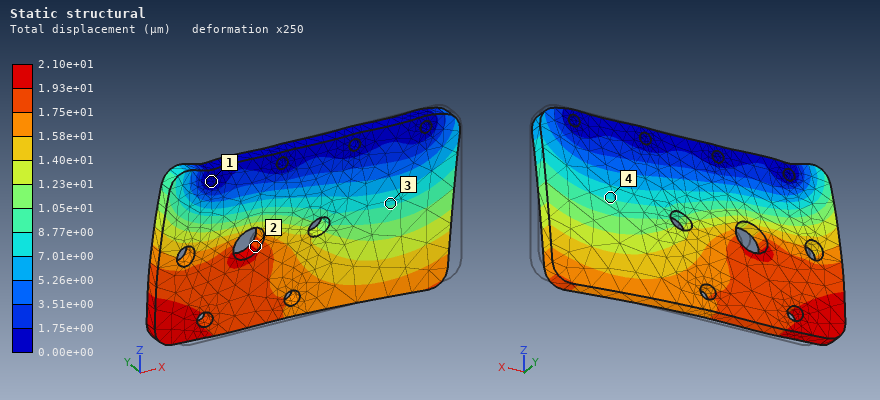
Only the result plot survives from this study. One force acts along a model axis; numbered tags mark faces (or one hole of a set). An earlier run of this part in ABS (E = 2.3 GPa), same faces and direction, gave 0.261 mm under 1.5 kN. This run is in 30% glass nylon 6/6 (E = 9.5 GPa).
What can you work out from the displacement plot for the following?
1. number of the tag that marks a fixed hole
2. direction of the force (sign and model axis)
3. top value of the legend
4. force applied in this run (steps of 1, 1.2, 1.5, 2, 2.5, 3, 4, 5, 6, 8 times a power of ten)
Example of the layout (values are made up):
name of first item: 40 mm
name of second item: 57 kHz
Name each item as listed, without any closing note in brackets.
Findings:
number of the tag that marks a fixed hole: 1
direction of the force: -X
top value of the legend: 2.10e+01 µm
force applied in this run: 500 N
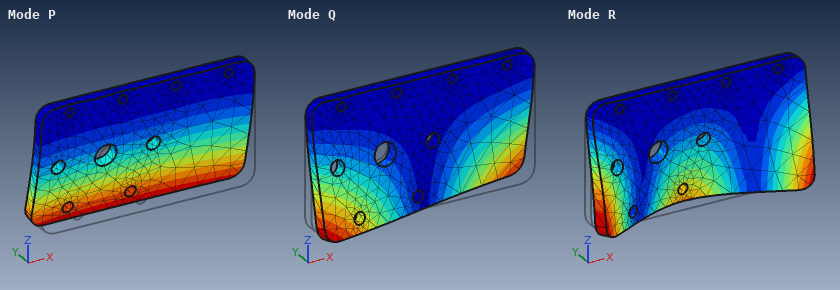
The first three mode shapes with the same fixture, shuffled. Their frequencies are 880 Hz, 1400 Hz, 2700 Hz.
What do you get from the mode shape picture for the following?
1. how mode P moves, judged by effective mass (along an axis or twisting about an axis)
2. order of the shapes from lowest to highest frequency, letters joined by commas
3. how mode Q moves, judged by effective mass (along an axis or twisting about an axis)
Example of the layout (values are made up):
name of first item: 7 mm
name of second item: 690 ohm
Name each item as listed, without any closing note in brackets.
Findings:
how mode P moves, judged by effective mass: along Y
order of the shapes from lowest to highest frequency, letters joined by commas: P, Q, R
how mode Q moves, judged by effective mass: twisting about Z
